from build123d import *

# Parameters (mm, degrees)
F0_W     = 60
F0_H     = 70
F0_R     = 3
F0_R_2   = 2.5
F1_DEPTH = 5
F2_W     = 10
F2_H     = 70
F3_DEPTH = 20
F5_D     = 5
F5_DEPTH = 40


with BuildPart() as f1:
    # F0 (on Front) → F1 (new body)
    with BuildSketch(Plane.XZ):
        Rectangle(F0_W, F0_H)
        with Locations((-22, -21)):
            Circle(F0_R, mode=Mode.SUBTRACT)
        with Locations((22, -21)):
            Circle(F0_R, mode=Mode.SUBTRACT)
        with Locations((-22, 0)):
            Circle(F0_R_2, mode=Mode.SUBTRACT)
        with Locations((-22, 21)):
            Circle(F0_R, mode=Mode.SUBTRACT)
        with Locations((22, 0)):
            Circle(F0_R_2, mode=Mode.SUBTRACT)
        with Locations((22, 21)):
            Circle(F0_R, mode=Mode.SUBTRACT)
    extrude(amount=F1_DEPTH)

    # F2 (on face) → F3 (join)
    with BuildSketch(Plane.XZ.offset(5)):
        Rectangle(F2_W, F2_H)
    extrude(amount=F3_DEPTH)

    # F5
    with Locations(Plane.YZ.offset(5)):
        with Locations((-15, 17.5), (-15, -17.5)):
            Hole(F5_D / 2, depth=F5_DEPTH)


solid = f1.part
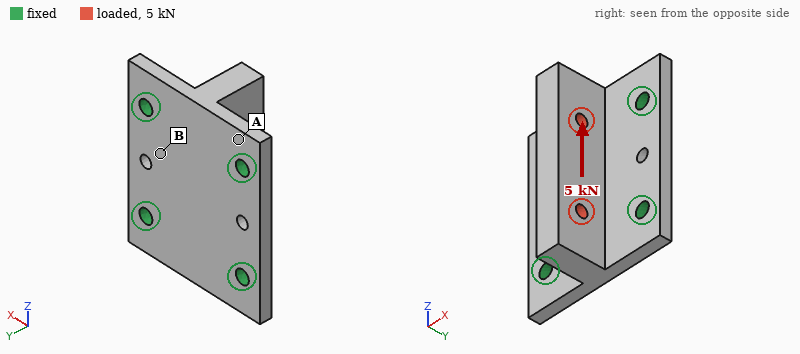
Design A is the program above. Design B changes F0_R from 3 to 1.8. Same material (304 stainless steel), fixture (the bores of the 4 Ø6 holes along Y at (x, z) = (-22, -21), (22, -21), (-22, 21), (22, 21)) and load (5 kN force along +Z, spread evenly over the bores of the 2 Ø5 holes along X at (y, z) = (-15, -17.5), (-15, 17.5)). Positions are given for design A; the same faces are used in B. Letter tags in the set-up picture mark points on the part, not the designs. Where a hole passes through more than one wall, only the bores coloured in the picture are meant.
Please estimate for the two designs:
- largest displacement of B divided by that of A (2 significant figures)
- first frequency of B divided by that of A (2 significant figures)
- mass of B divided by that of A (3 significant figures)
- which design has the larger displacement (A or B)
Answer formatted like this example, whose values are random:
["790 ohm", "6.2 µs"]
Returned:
["1.2", "0.88", "1.01", "B"]
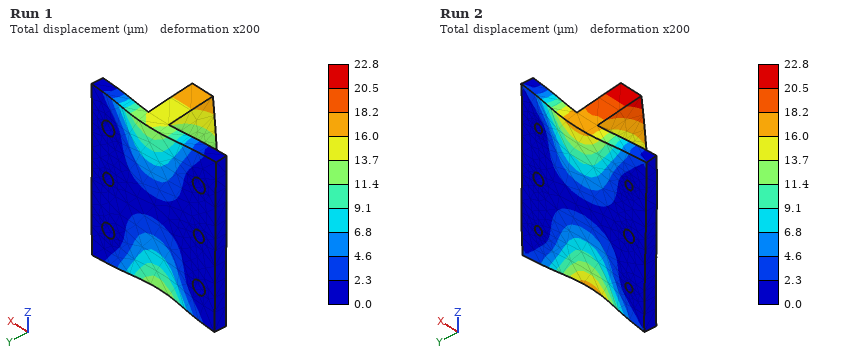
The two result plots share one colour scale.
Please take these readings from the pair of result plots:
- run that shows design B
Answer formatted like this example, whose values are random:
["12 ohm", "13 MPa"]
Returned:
["Run 2"]
